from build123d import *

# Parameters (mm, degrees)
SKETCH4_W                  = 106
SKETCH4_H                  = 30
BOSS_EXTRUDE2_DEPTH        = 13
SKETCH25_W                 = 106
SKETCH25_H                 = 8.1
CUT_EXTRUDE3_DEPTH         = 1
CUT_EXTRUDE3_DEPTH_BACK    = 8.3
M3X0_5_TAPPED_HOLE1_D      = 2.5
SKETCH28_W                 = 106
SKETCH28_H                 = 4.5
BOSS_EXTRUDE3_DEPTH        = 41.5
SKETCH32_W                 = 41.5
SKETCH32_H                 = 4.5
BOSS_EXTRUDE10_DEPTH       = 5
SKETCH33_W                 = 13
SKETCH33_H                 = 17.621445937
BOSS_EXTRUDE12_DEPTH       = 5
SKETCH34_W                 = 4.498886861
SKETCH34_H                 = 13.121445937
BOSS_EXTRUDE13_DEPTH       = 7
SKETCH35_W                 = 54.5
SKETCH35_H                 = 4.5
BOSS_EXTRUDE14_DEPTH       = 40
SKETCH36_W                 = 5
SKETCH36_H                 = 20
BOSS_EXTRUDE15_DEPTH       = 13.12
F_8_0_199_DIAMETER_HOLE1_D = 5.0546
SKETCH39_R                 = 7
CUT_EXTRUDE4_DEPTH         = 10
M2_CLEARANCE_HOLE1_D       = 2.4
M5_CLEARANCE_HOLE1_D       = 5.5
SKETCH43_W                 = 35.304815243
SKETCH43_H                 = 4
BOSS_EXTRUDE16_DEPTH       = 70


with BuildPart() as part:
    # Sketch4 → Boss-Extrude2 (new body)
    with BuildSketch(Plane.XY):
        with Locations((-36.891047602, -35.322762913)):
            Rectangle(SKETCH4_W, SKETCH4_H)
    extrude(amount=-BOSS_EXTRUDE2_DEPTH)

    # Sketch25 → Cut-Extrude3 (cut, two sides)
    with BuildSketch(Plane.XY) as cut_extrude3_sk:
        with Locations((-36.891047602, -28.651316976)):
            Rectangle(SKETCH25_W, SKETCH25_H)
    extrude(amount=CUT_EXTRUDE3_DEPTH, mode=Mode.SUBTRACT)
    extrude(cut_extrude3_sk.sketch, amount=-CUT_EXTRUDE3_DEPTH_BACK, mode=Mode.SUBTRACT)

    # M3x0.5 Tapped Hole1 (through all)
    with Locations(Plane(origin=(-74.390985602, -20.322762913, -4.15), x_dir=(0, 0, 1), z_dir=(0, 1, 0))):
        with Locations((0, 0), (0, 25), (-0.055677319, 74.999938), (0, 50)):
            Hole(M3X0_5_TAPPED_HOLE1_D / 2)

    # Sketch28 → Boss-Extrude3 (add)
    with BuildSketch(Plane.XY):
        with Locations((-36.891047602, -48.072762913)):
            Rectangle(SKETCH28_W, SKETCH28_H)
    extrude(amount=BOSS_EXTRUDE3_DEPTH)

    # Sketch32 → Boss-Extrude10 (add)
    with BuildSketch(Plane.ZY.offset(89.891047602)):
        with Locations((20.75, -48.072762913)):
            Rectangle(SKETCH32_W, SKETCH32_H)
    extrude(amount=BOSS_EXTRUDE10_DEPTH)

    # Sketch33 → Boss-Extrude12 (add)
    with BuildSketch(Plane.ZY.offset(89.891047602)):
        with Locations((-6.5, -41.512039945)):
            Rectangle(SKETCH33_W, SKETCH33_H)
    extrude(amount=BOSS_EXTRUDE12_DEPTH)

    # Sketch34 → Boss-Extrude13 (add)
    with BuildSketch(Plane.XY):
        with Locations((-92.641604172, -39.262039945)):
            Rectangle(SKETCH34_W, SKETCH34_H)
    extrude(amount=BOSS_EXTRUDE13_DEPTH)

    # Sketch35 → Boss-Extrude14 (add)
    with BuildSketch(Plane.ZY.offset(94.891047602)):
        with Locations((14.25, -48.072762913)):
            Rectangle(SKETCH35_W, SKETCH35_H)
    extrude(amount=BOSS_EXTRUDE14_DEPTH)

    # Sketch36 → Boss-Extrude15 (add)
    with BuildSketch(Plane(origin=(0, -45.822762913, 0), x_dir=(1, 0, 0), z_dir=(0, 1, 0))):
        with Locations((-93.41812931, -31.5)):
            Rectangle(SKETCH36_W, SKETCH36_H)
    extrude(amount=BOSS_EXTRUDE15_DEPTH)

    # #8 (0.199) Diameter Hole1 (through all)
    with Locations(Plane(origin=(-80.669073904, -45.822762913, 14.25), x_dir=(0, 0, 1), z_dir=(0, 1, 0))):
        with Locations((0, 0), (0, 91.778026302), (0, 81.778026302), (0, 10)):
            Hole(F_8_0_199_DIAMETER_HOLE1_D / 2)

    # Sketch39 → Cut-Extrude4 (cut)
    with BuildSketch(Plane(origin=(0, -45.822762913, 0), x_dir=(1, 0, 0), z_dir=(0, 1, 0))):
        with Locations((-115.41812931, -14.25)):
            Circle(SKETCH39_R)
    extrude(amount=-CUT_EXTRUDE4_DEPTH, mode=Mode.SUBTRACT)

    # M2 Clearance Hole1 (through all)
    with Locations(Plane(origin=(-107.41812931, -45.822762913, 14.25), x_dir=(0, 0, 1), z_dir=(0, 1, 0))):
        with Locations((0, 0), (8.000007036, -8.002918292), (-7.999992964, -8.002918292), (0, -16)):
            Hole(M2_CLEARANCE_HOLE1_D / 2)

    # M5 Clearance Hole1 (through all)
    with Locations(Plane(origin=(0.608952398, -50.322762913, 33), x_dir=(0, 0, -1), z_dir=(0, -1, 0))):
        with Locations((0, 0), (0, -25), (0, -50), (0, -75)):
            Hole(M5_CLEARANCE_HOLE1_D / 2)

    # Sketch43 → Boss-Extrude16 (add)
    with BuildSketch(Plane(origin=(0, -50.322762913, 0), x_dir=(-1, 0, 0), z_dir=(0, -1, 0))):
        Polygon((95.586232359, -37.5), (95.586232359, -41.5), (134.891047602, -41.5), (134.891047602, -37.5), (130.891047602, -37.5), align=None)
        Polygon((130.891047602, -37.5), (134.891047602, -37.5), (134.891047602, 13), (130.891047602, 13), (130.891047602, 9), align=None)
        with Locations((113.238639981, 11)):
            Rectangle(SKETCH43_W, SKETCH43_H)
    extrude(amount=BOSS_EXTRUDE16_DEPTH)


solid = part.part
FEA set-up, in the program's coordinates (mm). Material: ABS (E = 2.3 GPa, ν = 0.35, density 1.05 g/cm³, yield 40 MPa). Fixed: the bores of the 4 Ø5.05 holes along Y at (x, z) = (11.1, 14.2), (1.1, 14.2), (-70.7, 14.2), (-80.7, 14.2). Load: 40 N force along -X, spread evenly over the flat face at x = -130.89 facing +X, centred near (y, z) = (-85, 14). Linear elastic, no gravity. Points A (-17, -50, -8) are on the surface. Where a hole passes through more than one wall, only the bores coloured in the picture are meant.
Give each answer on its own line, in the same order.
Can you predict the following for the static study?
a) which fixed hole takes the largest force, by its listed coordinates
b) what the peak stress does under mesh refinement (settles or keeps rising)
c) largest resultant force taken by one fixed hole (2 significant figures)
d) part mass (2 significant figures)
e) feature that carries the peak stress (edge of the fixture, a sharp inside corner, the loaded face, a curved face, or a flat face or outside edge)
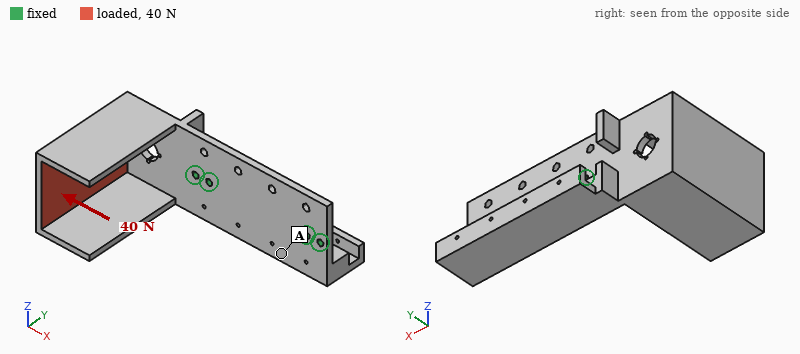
(-80.7, 14.2)
keeps rising
45 N
110 g
a sharp inside corner
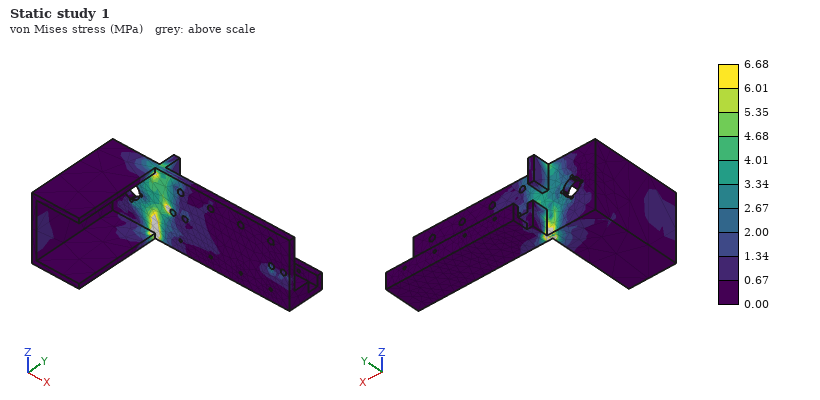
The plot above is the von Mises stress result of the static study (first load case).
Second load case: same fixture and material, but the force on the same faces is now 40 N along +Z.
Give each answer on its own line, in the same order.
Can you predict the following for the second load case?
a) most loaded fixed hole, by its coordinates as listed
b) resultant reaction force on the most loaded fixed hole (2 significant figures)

(-80.7, 14.2)
70 N
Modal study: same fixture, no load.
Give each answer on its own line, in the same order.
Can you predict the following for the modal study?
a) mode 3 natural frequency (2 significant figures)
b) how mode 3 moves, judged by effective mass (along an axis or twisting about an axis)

430 Hz
along Y
